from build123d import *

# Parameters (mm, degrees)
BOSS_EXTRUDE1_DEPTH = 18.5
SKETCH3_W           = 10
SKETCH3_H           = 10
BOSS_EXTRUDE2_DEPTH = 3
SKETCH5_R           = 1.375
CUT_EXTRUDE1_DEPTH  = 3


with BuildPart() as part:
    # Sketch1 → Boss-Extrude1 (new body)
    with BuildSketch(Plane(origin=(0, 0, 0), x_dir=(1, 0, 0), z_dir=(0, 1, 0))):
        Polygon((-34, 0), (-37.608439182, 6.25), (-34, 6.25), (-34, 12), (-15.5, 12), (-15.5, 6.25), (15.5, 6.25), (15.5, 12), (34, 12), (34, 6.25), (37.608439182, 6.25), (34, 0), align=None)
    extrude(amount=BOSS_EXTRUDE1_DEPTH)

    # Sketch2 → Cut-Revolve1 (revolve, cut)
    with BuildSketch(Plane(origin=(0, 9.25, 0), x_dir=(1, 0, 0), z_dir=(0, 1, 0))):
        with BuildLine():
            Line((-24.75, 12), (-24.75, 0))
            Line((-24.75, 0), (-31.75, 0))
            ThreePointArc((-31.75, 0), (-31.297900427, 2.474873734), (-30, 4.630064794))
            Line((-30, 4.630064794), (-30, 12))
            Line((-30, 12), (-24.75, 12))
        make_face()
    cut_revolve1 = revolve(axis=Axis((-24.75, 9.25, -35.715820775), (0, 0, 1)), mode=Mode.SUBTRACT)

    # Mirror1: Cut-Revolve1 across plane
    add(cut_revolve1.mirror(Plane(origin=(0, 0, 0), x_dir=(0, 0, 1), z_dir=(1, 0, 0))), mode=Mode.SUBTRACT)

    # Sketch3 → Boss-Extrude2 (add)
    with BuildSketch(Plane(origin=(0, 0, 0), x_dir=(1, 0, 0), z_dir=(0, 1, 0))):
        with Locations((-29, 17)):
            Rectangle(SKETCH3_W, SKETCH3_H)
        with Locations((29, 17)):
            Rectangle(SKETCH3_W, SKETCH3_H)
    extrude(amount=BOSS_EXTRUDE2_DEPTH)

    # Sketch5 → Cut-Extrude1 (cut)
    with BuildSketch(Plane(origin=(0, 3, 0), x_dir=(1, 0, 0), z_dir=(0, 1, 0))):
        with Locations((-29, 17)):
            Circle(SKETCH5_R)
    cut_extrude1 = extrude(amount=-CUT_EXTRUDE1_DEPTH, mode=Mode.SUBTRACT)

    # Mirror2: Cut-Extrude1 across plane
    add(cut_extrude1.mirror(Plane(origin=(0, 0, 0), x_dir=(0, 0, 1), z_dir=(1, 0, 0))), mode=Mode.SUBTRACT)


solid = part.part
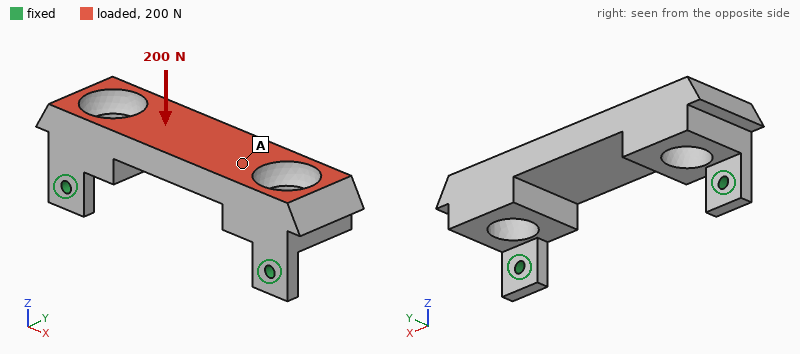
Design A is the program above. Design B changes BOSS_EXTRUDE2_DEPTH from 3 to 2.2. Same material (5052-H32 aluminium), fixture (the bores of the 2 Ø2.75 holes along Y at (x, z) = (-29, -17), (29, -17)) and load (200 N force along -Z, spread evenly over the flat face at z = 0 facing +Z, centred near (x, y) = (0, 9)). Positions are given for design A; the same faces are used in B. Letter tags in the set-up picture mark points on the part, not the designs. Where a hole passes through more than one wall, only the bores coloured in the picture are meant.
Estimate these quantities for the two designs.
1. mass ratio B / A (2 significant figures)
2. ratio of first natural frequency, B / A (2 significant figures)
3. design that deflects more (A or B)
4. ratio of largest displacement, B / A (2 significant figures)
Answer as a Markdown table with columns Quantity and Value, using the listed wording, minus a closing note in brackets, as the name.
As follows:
| Quantity | Value |
|---|---|
| mass ratio B / A | 0.99 |
| ratio of first natural frequency, B / A | 0.66 |
| design that deflects more | B |
| ratio of largest displacement, B / A | 2.3 |
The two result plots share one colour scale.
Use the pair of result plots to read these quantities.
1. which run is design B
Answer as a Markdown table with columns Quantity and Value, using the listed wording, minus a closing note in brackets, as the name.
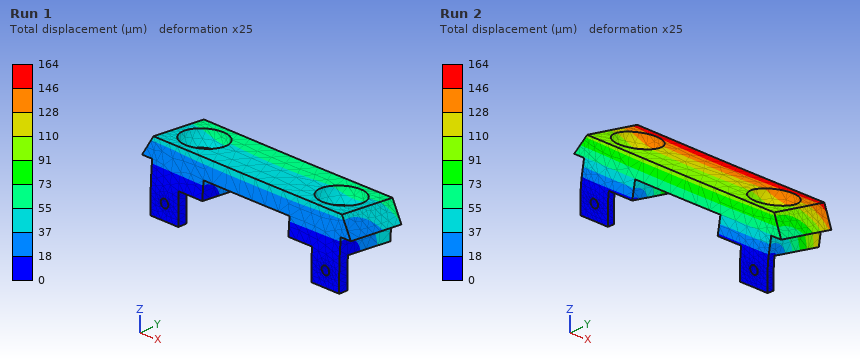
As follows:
| Quantity | Value |
|---|---|
| which run is design B | Run 2 |
